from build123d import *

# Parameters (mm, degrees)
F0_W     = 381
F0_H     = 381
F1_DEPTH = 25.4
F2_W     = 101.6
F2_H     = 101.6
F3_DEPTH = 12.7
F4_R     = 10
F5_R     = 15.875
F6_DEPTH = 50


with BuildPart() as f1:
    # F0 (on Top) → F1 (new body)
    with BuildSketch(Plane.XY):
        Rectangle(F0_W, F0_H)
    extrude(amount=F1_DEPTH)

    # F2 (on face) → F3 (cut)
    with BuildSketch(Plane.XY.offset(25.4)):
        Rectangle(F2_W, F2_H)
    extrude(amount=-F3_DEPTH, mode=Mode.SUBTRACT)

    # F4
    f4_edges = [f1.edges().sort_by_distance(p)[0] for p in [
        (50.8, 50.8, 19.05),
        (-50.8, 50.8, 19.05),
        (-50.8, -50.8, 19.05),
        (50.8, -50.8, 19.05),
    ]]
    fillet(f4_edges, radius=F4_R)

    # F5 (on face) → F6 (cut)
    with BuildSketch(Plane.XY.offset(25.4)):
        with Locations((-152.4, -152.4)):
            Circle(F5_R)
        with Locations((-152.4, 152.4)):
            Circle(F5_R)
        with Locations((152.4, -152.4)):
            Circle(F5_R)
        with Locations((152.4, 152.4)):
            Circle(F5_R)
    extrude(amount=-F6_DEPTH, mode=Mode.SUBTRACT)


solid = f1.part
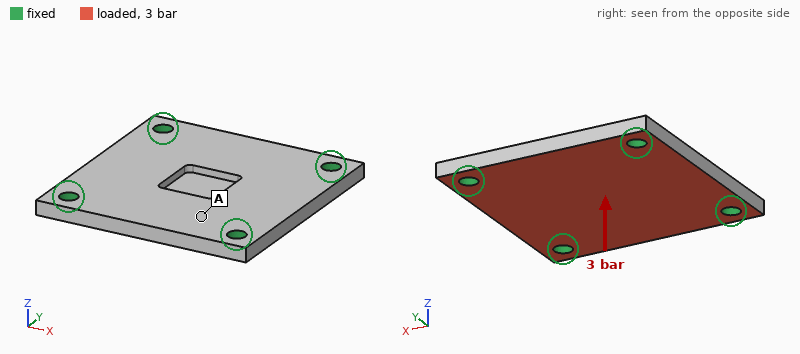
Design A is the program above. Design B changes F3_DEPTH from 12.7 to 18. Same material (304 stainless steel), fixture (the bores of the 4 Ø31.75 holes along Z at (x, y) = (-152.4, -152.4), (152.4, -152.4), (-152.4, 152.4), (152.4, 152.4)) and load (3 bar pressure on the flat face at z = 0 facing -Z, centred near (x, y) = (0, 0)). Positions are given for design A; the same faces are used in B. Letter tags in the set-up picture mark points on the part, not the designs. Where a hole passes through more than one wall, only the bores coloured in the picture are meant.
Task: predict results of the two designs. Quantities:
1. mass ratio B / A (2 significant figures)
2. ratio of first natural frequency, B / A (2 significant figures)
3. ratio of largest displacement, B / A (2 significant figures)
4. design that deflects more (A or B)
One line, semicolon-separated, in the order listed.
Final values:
0.98; 1.0; 1.1; B
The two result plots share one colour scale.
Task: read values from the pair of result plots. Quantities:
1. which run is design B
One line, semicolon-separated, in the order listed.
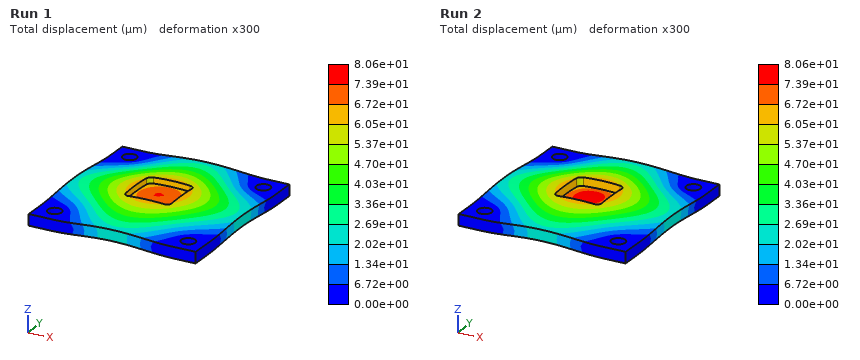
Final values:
Run 2
